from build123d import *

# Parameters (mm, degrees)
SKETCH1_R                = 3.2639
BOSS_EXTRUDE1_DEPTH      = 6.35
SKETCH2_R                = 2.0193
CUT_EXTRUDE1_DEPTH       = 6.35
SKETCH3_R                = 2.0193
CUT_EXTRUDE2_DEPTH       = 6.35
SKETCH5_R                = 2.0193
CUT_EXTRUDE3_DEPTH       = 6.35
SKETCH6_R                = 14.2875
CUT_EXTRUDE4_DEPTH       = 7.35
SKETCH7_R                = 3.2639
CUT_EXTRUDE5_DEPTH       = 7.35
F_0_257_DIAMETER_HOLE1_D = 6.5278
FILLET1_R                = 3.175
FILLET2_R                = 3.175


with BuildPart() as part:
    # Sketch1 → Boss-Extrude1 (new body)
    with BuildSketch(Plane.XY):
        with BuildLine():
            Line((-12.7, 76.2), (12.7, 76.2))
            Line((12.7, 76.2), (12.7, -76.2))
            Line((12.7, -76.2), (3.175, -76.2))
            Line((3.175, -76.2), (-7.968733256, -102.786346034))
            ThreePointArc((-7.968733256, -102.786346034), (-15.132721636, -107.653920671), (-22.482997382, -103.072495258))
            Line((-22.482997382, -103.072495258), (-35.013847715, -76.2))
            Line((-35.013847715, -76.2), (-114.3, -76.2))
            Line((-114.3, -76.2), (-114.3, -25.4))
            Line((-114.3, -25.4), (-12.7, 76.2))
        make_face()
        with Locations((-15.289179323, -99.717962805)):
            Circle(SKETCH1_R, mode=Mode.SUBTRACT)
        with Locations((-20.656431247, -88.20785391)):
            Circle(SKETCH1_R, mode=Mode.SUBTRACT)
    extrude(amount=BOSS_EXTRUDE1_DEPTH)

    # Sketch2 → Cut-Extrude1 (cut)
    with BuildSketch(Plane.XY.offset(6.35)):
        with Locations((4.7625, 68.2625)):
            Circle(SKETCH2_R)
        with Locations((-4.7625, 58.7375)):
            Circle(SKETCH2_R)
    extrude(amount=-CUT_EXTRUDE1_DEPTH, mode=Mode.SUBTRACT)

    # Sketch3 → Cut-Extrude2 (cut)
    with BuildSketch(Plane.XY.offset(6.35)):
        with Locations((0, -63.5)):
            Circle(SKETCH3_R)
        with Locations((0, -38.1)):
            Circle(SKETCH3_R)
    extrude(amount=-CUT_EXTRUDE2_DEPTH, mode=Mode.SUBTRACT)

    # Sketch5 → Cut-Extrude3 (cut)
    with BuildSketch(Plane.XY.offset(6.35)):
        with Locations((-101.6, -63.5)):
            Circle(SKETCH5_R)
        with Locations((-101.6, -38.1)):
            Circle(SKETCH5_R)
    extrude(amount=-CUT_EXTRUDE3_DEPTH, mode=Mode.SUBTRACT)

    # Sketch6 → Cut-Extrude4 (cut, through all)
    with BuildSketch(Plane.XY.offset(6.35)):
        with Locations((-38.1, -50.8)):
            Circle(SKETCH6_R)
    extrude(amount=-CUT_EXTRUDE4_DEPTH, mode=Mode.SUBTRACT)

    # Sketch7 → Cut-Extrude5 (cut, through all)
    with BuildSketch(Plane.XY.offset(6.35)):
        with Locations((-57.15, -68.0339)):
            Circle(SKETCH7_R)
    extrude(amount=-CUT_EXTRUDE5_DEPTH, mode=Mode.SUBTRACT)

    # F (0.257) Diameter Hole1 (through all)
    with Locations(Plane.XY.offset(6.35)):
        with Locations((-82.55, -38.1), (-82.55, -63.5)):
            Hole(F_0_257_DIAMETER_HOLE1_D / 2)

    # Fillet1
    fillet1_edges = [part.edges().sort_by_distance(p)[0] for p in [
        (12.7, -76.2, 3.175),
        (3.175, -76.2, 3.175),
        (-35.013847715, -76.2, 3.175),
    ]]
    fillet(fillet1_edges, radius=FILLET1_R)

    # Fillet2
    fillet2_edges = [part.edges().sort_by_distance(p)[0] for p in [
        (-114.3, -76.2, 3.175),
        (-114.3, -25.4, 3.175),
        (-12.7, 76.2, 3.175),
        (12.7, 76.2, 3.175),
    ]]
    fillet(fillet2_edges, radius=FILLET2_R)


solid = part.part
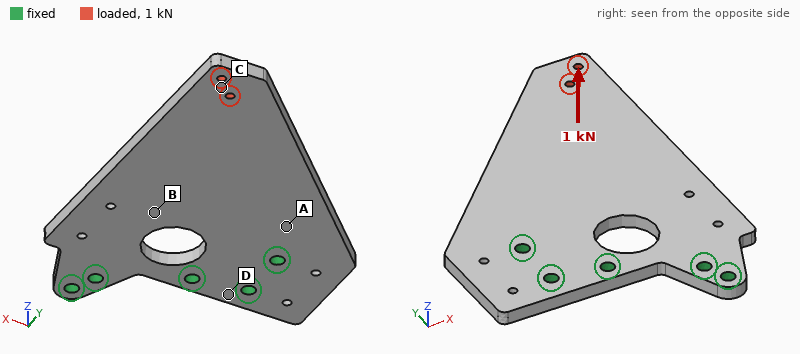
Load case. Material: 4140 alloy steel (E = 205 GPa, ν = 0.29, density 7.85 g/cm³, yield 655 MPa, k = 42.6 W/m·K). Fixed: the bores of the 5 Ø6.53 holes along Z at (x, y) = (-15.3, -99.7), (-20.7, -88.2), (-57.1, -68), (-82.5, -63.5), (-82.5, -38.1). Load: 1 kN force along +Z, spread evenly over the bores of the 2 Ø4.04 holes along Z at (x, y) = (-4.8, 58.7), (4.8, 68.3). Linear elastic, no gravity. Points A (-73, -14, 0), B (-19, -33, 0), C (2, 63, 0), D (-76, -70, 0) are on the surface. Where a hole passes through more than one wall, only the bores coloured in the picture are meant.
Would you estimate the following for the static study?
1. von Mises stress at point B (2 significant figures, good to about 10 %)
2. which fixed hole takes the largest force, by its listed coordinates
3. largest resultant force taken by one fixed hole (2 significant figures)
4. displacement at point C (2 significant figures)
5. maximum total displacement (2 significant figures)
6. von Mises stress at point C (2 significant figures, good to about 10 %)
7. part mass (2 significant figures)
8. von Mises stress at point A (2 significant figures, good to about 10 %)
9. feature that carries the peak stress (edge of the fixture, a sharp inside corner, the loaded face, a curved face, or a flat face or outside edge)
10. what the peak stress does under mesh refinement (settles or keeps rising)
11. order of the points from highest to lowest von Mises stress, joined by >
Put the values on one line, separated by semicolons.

100 MPa; (-82.5, -38.1); 2.1 kN; 2.0 mm; 2.4 mm; 50 MPa; 700 g; 160 MPa; edge of the fixture; keeps rising; A > B > C > D
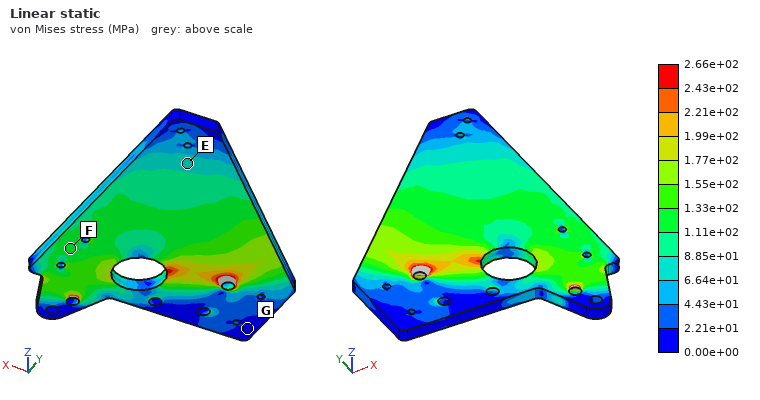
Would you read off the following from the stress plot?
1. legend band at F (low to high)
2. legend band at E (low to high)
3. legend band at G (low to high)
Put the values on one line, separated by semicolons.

1.11e+02 to 1.33e+02 MPa; 6.64e+01 to 8.85e+01 MPa; 0.00e+00 to 2.21e+01 MPa
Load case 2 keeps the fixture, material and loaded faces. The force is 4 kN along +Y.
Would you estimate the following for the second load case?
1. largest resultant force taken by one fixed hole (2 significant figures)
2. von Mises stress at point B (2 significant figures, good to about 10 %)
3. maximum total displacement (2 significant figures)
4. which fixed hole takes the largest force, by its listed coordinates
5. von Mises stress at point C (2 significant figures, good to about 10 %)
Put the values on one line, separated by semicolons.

2.4 kN; 15 MPa; 28 µm; (-20.7, -88.2); 26 MPa
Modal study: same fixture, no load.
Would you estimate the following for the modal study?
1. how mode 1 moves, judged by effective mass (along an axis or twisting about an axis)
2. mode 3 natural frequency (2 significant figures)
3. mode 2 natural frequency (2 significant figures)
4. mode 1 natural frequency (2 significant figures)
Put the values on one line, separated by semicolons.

along Z; 1800 Hz; 1400 Hz; 350 Hz
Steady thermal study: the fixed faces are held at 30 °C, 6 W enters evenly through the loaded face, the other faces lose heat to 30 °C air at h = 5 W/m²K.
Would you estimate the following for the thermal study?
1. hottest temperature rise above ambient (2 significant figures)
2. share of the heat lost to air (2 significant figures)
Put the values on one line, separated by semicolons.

42 K; 27 %
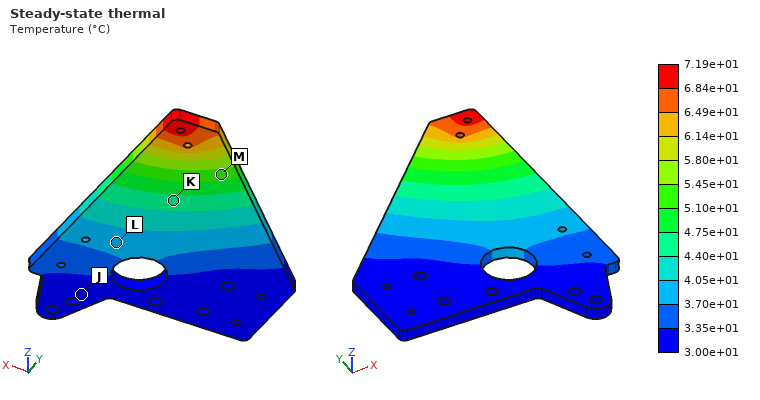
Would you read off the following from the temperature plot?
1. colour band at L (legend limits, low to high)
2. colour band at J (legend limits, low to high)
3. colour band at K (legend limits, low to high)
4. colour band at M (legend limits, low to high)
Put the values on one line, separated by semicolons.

3.70e+01 to 4.05e+01 °C; 3.00e+01 to 3.35e+01 °C; 4.40e+01 to 4.75e+01 °C; 5.10e+01 to 5.45e+01 °C
